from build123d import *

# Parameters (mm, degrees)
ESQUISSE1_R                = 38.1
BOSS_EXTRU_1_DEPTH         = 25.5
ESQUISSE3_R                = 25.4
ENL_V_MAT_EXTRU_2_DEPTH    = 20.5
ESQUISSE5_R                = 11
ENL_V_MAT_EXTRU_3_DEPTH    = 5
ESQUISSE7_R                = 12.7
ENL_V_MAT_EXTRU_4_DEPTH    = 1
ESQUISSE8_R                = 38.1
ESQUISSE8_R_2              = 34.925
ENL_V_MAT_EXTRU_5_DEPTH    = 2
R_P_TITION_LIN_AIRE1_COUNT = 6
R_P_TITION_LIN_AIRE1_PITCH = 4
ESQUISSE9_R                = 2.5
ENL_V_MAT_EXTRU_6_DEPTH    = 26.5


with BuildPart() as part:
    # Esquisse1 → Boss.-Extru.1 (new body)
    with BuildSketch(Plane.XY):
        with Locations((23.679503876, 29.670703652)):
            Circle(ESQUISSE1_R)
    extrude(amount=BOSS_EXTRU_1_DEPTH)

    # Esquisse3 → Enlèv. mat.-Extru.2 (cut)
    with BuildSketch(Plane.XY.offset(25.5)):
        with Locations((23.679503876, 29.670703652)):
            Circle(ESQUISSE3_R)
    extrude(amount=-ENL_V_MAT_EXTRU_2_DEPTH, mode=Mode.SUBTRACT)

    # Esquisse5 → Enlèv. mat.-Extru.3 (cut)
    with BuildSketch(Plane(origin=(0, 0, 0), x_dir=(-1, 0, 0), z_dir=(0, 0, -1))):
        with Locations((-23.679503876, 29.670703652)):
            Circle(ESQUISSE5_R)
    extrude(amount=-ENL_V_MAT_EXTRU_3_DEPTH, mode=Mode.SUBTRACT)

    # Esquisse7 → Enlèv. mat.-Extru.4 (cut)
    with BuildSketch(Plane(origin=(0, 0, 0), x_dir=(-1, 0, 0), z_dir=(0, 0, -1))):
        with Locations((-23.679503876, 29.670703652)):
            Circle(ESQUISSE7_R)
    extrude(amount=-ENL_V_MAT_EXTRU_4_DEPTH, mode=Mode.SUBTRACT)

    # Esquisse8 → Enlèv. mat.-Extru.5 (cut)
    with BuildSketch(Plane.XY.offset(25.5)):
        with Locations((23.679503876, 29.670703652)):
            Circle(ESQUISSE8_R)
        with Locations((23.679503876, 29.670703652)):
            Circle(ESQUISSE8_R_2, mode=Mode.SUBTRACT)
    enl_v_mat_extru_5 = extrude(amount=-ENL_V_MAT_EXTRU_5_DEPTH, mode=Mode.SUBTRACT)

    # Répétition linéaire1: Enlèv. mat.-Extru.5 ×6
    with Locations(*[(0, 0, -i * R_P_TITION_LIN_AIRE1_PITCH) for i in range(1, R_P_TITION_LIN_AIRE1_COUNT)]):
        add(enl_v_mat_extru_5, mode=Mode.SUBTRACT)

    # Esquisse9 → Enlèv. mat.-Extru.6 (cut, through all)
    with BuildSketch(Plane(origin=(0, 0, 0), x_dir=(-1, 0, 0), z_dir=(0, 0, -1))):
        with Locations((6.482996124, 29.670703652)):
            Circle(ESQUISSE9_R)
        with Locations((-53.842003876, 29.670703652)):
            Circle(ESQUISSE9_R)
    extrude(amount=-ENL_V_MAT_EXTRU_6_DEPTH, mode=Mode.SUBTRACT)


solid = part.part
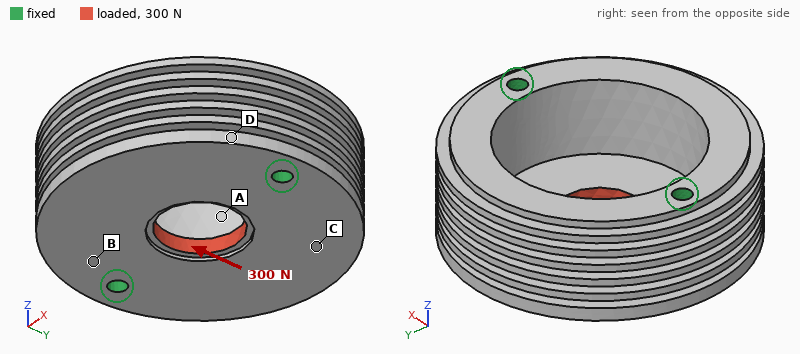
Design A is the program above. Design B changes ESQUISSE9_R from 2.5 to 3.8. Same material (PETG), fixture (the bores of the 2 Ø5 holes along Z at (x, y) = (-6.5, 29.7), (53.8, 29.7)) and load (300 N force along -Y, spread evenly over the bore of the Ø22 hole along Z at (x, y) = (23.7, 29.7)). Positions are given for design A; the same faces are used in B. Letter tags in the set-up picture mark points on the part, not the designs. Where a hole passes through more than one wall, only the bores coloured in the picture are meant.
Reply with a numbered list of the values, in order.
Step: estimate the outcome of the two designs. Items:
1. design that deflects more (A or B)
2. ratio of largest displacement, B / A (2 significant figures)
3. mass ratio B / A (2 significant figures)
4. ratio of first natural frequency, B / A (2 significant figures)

1. A
2. 0.89
3. 0.98
4. 1.1
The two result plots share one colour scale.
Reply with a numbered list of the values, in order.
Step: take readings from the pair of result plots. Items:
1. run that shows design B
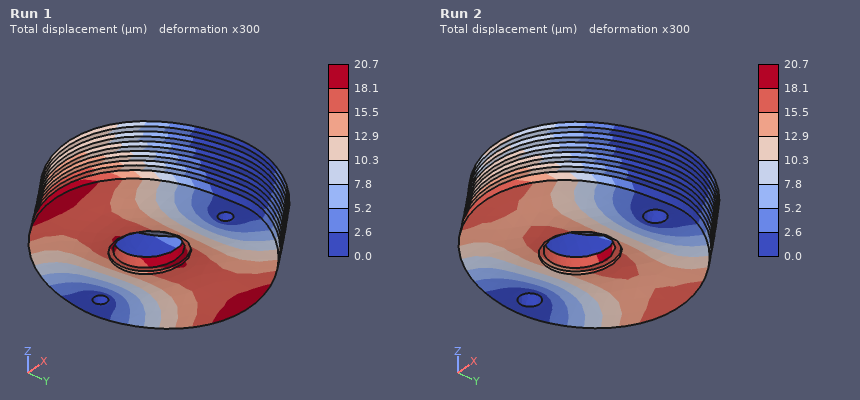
1. Run 2
